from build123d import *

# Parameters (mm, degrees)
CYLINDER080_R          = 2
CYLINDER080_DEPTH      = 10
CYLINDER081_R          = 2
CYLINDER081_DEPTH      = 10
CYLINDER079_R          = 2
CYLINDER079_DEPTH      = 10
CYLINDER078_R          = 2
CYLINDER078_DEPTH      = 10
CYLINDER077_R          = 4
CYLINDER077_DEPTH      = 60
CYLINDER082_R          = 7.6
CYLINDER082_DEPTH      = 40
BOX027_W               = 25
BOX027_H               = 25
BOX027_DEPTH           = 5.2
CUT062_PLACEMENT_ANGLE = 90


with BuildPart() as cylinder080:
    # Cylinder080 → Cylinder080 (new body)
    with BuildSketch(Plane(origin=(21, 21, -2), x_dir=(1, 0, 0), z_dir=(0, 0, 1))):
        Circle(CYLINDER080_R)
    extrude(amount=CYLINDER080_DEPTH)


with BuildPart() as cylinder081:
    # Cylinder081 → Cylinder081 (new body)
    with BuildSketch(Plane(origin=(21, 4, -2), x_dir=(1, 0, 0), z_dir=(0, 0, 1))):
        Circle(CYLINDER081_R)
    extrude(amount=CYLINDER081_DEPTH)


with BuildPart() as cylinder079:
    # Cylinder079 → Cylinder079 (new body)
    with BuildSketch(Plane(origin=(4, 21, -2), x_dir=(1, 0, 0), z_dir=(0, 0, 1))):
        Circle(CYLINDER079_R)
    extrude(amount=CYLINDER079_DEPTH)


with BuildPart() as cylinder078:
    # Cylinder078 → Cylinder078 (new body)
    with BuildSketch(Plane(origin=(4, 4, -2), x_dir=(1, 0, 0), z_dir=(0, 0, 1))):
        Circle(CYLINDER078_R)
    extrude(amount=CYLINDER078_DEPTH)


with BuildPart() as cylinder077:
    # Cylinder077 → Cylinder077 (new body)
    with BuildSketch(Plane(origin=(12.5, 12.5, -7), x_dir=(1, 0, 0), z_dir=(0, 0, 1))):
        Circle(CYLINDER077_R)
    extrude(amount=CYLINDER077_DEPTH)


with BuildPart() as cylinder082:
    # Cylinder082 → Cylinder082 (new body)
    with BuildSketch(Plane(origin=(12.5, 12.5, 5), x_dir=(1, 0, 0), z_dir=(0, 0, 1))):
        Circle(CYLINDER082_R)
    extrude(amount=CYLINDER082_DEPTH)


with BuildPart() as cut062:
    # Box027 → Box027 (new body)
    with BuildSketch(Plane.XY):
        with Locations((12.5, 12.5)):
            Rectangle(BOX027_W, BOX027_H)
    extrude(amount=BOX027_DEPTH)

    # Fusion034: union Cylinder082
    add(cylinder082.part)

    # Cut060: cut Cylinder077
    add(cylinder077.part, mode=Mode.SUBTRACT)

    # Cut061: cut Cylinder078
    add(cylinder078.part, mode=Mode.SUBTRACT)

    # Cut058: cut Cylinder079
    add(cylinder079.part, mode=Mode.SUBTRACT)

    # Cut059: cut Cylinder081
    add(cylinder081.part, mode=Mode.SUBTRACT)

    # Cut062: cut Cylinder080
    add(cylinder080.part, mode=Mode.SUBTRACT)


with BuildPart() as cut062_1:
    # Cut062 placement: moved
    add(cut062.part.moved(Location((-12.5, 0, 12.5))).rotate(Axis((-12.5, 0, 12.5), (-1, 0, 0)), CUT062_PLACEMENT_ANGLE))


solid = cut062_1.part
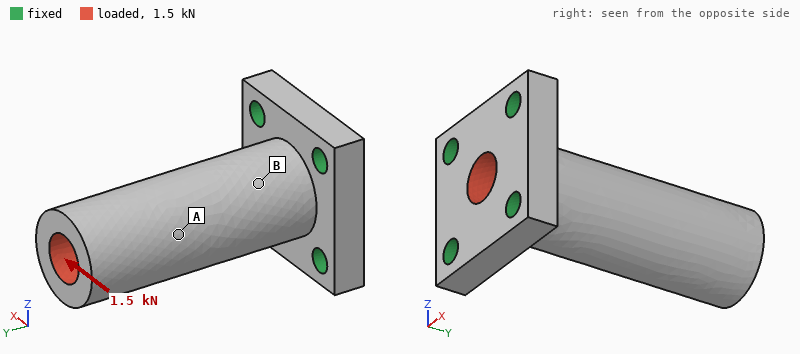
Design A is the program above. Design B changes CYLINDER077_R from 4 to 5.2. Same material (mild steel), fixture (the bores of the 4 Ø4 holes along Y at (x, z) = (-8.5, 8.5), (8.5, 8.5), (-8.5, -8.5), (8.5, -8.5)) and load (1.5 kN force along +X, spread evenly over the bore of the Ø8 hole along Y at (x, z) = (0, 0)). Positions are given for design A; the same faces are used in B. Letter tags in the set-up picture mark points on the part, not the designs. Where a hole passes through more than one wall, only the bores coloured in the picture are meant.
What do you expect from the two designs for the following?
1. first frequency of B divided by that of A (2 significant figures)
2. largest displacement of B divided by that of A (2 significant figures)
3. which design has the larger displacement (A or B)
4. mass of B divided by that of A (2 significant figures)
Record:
1.1
1.2
B
0.80
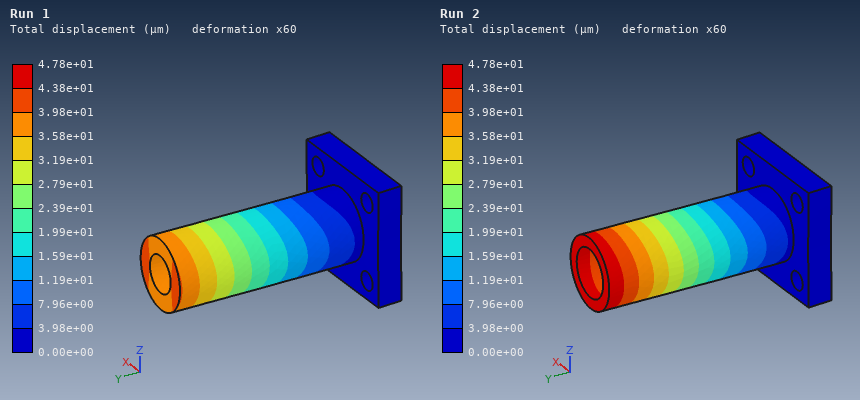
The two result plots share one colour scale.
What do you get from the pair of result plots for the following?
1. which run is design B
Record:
Run 2
